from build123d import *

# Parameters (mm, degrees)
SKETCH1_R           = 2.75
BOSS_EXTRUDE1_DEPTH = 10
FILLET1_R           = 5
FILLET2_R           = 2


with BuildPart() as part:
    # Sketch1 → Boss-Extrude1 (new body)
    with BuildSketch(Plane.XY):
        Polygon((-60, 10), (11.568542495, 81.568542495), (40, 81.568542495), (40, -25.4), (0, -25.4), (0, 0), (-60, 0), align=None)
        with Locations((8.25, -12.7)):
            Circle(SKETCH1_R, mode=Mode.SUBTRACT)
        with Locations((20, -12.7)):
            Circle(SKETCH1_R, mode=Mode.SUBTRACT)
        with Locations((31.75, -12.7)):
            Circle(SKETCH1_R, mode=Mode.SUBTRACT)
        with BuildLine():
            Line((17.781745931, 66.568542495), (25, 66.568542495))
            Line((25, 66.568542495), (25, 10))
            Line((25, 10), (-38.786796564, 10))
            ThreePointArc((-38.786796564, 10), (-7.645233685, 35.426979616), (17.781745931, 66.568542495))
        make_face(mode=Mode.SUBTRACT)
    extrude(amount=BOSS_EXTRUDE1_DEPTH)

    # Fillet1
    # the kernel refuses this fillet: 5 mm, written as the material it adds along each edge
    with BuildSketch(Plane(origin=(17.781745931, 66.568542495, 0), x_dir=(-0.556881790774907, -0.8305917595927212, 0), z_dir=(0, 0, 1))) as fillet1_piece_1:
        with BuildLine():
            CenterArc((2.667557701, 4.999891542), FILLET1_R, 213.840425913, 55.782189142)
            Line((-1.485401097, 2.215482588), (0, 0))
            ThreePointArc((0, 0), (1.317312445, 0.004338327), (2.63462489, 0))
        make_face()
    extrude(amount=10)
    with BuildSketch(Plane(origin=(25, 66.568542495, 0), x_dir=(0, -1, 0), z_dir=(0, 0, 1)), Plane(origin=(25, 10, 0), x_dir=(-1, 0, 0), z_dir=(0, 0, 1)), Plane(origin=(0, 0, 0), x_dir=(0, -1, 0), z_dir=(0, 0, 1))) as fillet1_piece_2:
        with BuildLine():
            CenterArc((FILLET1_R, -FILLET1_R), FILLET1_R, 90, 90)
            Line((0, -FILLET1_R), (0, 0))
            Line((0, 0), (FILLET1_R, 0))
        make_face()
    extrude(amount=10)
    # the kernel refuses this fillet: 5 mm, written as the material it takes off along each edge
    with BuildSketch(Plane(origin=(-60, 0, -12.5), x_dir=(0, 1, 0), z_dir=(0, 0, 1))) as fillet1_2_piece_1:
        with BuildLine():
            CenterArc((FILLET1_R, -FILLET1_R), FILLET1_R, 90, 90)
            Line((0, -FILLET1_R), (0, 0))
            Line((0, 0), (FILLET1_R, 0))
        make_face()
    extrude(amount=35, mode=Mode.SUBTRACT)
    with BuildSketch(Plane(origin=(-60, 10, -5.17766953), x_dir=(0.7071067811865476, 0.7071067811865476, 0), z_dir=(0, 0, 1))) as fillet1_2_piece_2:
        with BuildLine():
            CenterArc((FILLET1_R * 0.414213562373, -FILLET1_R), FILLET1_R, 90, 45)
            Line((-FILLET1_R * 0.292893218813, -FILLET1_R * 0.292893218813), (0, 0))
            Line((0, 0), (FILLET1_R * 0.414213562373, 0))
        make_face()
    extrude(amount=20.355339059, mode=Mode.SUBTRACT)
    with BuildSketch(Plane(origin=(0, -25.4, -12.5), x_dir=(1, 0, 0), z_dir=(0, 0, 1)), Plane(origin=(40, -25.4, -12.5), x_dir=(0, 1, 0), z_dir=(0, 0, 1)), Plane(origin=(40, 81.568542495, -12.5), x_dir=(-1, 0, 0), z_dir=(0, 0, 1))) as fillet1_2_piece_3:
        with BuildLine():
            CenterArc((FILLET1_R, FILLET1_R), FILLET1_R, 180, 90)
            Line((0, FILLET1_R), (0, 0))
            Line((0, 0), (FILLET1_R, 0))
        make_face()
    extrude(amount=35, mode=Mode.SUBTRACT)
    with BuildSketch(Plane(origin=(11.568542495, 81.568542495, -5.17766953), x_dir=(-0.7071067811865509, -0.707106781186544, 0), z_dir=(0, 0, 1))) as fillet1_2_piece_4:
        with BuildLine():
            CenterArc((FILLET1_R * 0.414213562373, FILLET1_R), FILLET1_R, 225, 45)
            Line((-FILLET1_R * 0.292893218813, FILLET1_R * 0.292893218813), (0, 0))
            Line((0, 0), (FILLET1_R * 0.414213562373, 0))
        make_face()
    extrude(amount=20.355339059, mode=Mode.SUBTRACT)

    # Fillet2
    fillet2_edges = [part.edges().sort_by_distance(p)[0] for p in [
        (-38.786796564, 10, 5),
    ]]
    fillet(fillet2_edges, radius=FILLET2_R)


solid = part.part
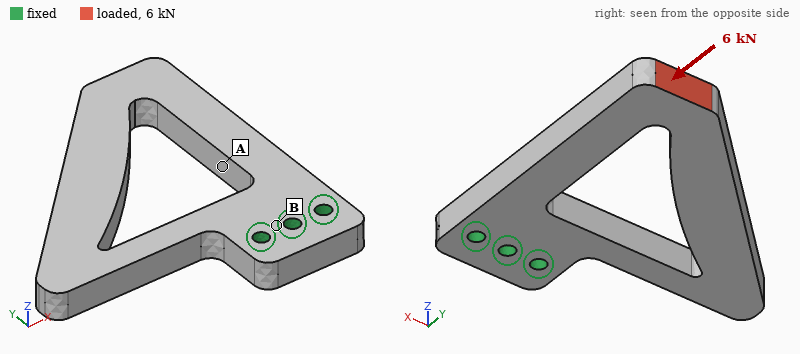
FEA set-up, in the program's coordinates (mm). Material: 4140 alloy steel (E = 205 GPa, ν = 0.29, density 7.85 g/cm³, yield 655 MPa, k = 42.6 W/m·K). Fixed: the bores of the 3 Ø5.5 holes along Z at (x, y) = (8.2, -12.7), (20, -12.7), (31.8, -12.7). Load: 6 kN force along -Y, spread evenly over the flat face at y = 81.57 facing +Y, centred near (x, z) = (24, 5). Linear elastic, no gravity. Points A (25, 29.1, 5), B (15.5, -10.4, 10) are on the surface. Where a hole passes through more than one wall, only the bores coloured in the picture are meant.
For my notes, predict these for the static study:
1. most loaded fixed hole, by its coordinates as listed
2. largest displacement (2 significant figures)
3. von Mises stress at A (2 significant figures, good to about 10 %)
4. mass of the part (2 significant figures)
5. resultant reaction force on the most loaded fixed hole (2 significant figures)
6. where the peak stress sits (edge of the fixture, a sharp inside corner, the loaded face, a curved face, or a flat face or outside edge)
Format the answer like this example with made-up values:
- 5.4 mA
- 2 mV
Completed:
- (31.8, -12.7)
- 62 µm
- 64 MPa
- 370 g
- 3.4 kN
- a curved face
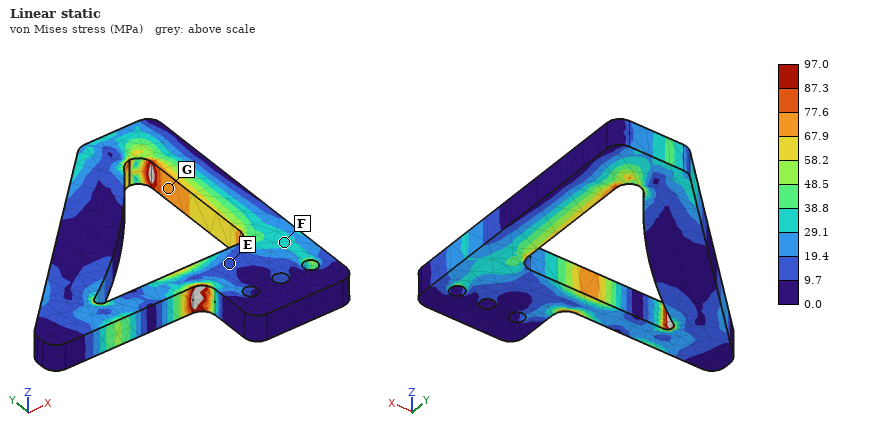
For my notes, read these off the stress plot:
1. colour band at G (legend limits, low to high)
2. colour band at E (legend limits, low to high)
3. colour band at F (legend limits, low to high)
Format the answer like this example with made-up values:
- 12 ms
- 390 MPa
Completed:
- 67.9 to 77.6 MPa
- 9.7 to 19.4 MPa
- 29.1 to 38.8 MPa
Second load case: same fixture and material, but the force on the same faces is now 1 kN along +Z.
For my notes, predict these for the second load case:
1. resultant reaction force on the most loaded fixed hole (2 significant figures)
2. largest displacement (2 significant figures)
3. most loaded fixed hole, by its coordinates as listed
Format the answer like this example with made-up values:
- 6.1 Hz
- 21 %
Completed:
- 930 N
- 0.65 mm
- (20, -12.7)
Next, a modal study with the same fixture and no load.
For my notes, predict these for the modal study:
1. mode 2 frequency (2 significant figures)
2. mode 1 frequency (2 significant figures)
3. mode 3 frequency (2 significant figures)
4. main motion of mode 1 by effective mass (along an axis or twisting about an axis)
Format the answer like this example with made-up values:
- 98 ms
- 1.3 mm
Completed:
- 1200 Hz
- 740 Hz
- 1400 Hz
- along Z
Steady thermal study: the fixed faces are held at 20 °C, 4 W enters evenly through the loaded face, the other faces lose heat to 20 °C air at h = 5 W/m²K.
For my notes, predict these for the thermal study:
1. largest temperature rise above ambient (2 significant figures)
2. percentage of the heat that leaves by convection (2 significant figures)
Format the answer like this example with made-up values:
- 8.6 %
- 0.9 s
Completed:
- 30 K
- 23 %
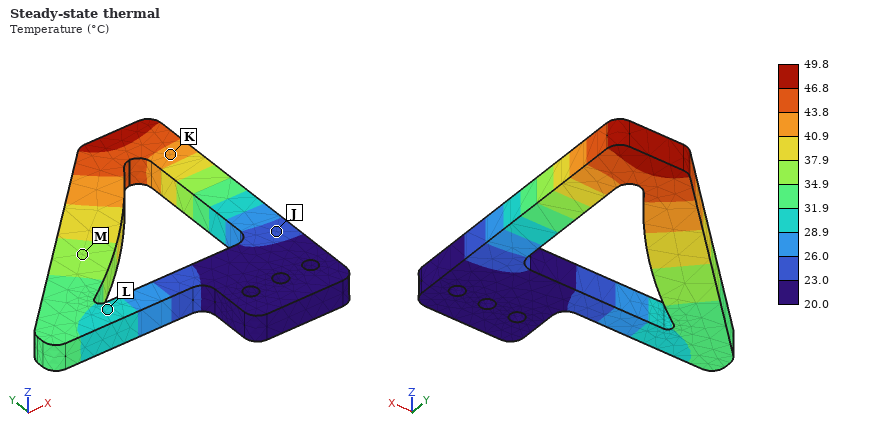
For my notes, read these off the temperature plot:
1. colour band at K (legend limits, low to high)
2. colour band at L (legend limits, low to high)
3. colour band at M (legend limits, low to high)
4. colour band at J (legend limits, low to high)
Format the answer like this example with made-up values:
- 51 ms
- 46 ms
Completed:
- 40.9 to 43.8 °C
- 28.9 to 31.9 °C
- 34.9 to 37.9 °C
- 23.0 to 26.0 °C
